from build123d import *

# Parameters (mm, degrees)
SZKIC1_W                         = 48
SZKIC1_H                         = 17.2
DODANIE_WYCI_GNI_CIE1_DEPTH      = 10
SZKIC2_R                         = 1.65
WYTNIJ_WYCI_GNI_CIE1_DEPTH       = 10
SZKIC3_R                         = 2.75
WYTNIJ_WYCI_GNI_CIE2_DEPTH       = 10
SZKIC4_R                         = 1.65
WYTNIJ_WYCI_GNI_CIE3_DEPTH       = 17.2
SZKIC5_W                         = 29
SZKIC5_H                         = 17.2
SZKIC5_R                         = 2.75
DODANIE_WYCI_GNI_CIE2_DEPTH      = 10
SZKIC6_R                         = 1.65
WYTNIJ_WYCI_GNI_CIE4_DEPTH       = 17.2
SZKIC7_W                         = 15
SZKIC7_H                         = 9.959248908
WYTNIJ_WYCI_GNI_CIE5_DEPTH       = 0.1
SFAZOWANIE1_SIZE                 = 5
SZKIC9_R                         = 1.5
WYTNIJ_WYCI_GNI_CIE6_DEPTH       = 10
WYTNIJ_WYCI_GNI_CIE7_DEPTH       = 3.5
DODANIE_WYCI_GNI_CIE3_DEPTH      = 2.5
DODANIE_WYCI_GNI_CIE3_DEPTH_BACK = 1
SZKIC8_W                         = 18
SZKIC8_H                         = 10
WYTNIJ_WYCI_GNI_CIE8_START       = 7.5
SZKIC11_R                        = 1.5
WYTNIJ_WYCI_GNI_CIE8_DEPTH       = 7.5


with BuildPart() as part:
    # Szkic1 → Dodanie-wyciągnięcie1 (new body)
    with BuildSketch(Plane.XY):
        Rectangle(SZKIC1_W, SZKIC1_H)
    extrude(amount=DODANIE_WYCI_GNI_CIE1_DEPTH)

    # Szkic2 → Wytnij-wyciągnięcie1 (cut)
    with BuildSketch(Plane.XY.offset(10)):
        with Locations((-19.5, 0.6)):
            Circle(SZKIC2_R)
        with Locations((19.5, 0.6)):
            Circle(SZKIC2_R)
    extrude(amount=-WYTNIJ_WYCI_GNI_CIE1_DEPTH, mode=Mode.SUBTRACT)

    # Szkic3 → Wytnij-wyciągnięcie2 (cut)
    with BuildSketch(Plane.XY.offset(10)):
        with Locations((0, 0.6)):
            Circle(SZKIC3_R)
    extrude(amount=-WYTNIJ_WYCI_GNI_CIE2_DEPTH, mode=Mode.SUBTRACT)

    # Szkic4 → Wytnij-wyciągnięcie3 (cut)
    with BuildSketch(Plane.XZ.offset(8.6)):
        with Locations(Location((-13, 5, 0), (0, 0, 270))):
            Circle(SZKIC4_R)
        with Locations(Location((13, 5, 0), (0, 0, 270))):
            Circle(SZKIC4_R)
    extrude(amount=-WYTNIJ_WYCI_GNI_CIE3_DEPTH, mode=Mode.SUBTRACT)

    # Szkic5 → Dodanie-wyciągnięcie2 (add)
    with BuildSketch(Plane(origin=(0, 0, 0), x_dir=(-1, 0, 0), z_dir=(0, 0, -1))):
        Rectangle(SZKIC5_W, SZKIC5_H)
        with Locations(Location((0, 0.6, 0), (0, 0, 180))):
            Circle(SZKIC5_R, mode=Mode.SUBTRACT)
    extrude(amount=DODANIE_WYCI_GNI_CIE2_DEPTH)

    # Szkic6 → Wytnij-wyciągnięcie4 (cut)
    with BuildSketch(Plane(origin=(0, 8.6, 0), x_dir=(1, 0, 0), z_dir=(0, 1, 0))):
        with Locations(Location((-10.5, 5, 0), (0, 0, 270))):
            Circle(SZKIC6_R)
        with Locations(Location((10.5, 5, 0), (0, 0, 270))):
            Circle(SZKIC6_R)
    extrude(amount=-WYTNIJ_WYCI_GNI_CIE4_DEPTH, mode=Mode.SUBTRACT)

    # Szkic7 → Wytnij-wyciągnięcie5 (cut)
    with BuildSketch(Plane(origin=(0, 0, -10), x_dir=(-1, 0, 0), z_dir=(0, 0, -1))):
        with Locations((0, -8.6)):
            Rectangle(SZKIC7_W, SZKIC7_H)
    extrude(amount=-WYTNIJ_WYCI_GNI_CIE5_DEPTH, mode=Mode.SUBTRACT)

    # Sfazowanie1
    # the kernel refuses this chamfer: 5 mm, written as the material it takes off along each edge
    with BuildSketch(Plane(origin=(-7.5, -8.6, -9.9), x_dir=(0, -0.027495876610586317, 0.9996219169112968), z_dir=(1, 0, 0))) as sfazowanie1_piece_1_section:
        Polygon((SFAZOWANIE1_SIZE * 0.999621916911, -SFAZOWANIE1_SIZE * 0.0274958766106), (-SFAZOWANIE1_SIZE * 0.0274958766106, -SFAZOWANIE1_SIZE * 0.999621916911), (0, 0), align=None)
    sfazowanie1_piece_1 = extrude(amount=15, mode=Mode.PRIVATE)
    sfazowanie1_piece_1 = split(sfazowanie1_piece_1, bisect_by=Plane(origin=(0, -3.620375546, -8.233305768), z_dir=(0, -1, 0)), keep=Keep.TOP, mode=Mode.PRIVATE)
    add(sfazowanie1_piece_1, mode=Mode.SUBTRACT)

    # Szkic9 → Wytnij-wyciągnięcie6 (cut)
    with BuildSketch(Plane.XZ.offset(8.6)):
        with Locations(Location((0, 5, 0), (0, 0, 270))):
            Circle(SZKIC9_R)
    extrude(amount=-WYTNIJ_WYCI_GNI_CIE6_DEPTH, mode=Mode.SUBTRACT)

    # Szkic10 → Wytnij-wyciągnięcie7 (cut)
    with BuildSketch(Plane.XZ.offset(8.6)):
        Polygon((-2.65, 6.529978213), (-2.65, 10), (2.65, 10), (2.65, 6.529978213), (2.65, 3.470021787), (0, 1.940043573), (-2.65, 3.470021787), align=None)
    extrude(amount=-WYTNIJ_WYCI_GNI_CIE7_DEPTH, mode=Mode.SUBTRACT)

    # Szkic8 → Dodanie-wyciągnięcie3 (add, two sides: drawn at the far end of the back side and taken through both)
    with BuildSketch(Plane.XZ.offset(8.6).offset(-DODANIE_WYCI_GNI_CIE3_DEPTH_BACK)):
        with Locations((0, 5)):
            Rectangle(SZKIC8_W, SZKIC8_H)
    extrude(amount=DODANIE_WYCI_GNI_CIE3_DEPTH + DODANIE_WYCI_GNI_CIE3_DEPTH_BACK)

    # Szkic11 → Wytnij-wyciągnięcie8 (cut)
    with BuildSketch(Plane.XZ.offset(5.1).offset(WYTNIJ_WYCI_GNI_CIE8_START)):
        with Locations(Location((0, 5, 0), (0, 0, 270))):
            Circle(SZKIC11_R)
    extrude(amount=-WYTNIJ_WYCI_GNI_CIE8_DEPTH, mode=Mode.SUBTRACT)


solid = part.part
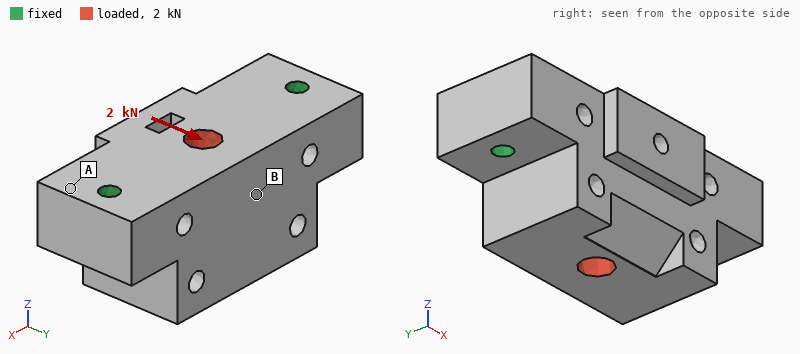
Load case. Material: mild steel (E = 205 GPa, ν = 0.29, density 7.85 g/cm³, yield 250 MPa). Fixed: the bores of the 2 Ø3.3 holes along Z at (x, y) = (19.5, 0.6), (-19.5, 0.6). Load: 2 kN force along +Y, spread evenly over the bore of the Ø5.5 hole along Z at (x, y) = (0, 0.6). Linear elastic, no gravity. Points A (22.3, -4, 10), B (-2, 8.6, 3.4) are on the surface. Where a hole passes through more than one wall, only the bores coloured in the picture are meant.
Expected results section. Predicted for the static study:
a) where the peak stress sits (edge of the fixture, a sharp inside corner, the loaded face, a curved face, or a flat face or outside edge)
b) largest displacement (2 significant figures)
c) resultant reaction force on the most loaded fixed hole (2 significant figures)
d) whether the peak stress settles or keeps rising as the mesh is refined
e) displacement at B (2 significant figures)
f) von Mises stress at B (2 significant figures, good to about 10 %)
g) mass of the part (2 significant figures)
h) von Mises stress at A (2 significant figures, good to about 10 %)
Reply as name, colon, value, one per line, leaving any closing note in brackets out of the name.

where the peak stress sits: edge of the fixture
largest displacement: 5.6 µm
resultant reaction force on the most loaded fixed hole: 1.0 kN
whether the peak stress settles or keeps rising as the mesh is refined: keeps rising
displacement at B: 3.0 µm
von Mises stress at B: 17 MPa
mass of the part: 95 g
von Mises stress at A: 6.5 MPa
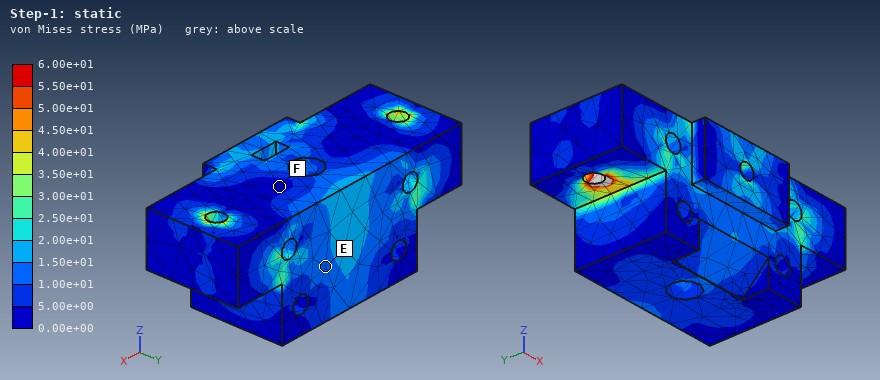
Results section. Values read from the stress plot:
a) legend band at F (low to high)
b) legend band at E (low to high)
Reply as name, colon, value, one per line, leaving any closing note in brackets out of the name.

legend band at F: 0.00e+00 to 5.00e+00 MPa
legend band at E: 1.00e+01 to 1.50e+01 MPa
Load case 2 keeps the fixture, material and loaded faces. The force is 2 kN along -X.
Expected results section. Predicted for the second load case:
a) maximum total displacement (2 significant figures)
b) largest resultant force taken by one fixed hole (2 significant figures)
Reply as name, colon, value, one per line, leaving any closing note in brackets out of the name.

maximum total displacement: 1.0 µm
largest resultant force taken by one fixed hole: 1.0 kN
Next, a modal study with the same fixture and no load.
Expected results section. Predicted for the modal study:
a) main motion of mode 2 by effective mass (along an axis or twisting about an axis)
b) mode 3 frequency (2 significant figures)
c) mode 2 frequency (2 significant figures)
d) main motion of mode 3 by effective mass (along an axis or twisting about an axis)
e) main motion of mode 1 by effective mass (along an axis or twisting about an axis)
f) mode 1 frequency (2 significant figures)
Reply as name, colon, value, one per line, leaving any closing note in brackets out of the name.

main motion of mode 2 by effective mass: along Z
mode 3 frequency: 25 kHz
mode 2 frequency: 21 kHz
main motion of mode 3 by effective mass: along Y
main motion of mode 1 by effective mass: along Y
mode 1 frequency: 14 kHz
